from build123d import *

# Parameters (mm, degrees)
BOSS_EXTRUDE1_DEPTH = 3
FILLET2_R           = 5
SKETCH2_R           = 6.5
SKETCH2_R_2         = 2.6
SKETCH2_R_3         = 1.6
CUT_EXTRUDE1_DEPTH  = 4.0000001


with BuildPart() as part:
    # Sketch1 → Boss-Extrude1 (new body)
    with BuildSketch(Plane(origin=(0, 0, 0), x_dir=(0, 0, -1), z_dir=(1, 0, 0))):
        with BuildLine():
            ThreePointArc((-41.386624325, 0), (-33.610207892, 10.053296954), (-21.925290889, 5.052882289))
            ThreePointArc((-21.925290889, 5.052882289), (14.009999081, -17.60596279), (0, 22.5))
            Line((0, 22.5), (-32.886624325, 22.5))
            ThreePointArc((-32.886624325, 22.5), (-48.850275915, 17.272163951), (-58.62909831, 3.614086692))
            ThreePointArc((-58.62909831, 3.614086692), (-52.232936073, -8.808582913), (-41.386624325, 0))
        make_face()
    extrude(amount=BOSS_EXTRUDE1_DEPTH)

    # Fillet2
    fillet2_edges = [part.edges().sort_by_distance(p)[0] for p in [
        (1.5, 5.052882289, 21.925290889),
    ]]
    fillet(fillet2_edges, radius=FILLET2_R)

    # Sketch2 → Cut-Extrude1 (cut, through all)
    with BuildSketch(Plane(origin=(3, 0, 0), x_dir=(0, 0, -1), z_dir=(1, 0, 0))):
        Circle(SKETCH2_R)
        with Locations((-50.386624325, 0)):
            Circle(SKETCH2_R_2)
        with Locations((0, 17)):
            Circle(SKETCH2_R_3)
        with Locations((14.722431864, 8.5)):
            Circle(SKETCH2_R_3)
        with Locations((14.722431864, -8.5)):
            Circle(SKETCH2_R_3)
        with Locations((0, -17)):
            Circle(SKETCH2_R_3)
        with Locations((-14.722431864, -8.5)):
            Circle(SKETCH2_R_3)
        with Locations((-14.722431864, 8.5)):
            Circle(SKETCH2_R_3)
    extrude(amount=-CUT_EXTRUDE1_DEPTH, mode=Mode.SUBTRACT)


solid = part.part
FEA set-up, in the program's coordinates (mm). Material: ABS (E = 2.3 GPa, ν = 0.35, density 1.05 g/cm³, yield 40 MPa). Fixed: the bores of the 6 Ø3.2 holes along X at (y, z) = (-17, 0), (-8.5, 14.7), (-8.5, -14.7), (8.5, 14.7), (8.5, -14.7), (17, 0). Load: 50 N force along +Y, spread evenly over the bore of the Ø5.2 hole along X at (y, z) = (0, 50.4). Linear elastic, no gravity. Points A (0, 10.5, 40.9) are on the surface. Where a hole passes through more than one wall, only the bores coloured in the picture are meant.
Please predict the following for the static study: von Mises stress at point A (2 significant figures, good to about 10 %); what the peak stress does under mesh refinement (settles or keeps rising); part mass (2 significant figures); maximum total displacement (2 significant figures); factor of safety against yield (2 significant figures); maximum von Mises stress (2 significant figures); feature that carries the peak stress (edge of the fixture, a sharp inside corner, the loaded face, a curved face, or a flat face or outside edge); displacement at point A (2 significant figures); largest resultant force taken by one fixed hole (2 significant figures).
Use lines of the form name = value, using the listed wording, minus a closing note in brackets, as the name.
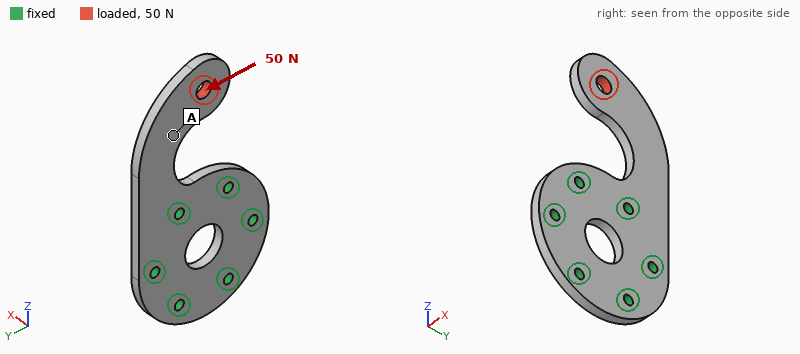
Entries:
von Mises stress at point A = 3.1 MPa
what the peak stress does under mesh refinement = settles
part mass = 6.8 g
maximum total displacement = 0.85 mm
factor of safety against yield = 2.1
maximum von Mises stress = 19 MPa
feature that carries the peak stress = a curved face
displacement at point A = 0.33 mm
largest resultant force taken by one fixed hole = 79 N
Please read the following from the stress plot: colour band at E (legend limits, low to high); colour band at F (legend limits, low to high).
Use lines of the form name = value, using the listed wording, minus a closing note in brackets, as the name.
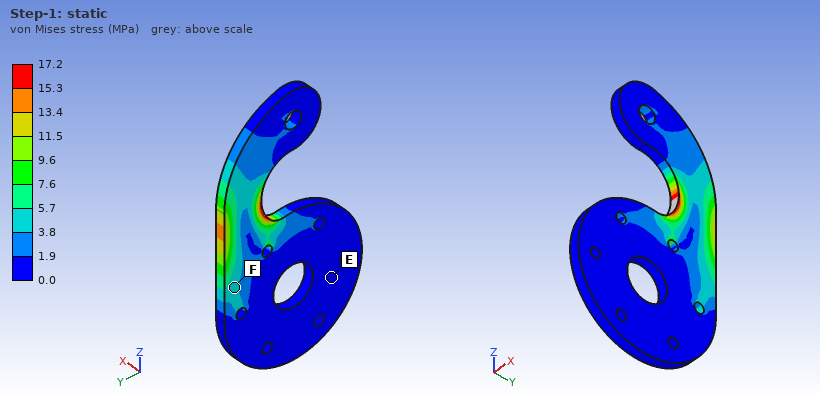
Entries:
colour band at E = 0.0 to 1.9 MPa
colour band at F = 3.8 to 5.7 MPa
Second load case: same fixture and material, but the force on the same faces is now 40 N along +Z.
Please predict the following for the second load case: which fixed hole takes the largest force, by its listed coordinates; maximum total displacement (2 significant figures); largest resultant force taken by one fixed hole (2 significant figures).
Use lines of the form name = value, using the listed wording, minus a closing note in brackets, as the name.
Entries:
which fixed hole takes the largest force, by its listed coordinates = (8.5, 14.7)
maximum total displacement = 0.49 mm
largest resultant force taken by one fixed hole = 44 N
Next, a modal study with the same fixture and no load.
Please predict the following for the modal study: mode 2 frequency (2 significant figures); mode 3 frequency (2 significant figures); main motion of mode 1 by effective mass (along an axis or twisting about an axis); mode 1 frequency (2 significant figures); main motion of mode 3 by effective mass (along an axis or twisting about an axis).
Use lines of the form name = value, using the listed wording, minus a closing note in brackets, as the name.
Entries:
mode 2 frequency = 950 Hz
mode 3 frequency = 1200 Hz
main motion of mode 1 by effective mass = along X
mode 1 frequency = 310 Hz
main motion of mode 3 by effective mass = along Y
